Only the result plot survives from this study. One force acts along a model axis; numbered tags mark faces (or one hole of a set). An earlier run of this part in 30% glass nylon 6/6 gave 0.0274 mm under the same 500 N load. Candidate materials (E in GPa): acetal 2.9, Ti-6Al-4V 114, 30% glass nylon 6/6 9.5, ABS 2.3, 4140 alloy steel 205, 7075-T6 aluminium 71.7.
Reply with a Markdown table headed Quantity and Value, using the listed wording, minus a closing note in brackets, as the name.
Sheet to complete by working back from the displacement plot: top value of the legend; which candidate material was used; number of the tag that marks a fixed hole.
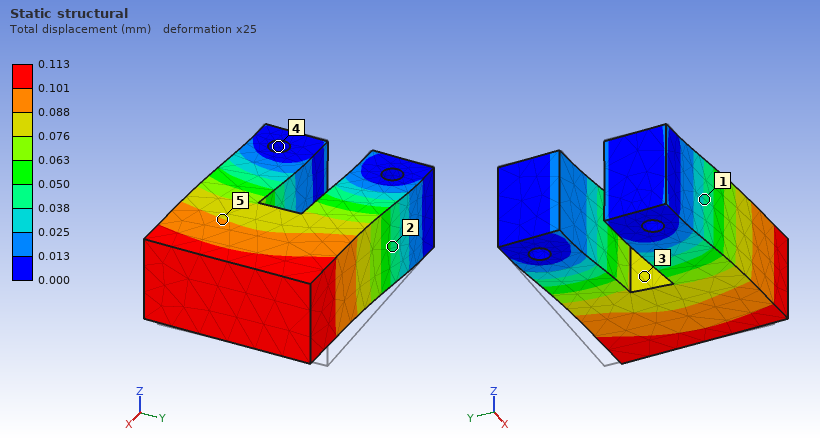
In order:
| Quantity | Value |
|---|---|
| top value of the legend | 0.113 mm |
| which candidate material was used | ABS |
| number of the tag that marks a fixed hole | 4 |
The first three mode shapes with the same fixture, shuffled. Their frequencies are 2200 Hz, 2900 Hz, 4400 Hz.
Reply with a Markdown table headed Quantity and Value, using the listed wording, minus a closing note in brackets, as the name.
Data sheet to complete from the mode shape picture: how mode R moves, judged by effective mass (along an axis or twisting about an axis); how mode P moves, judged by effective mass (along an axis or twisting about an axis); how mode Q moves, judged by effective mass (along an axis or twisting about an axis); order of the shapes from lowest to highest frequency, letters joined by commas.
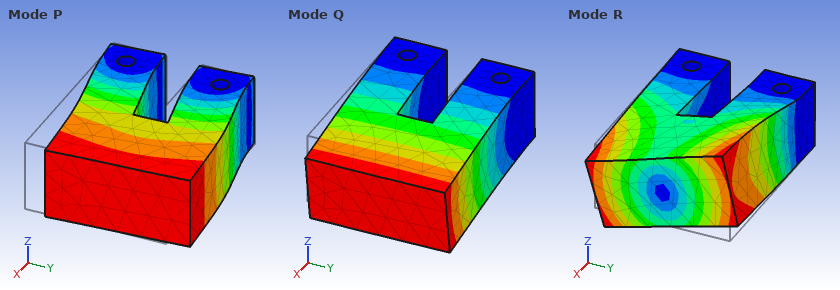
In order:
| Quantity | Value |
|---|---|
| how mode R moves, judged by effective mass | twisting about X |
| how mode P moves, judged by effective mass | along Y |
| how mode Q moves, judged by effective mass | along Z |
| order of the shapes from lowest to highest frequency, letters joined by commas | Q, P, R |
